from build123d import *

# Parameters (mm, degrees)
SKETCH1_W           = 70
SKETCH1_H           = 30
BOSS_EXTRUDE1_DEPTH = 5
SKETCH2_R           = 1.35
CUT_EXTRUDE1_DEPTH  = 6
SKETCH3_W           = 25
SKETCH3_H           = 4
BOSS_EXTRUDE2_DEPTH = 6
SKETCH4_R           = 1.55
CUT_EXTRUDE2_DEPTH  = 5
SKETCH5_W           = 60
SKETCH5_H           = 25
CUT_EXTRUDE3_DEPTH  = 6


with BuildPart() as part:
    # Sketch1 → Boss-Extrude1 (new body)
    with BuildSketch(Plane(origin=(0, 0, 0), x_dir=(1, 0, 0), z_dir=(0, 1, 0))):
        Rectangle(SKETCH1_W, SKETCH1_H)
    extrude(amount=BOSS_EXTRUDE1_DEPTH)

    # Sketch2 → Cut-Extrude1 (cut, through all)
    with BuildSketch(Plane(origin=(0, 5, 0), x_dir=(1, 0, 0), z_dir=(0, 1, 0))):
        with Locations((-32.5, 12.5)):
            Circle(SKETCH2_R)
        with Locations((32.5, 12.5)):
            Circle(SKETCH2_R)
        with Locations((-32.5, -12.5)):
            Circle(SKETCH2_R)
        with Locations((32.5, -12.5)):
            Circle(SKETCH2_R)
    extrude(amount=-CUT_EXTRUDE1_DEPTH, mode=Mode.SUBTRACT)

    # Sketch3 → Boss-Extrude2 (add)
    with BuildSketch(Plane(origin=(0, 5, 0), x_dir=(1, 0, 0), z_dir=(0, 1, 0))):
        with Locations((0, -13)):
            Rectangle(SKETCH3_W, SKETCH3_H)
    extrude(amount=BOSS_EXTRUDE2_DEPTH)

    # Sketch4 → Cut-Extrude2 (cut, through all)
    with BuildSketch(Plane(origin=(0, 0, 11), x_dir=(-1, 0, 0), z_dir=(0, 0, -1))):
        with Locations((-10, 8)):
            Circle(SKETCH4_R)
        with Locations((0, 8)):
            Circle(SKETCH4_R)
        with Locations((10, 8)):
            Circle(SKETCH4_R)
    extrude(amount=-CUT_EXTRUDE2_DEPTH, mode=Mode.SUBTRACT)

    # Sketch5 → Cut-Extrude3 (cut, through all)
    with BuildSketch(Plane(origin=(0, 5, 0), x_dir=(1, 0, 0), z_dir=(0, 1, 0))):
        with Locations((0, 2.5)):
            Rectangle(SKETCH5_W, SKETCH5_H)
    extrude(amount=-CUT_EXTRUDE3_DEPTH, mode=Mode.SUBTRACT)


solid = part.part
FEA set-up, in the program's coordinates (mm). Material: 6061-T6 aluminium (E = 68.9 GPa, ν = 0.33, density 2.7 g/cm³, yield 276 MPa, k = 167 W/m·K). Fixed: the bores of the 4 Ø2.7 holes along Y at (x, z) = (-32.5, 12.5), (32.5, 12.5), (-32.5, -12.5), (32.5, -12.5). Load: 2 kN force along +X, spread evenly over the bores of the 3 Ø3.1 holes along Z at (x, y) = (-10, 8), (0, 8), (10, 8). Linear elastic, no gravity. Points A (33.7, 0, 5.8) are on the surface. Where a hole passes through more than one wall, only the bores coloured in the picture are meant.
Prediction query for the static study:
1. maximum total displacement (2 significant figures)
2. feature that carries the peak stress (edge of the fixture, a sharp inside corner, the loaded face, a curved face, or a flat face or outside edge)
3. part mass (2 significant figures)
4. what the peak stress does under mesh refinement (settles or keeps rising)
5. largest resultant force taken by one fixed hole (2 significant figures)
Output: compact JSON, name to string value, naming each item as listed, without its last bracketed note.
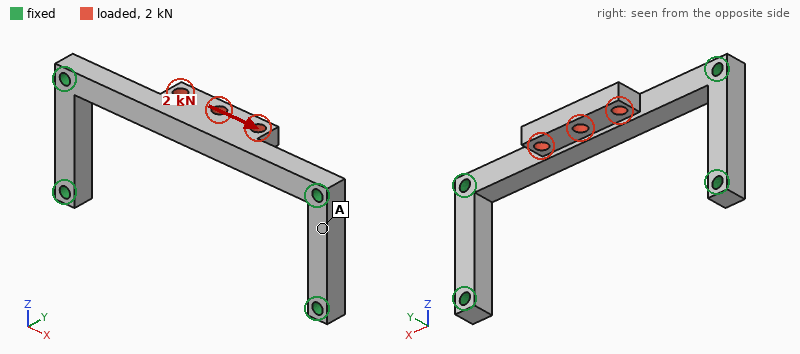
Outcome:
{"maximum total displacement": "56 µm", "feature that carries the peak stress": "edge of the fixture", "part mass": "9.2 g", "what the peak stress does under mesh refinement": "keeps rising", "largest resultant force taken by one fixed hole": "1.0 kN"}
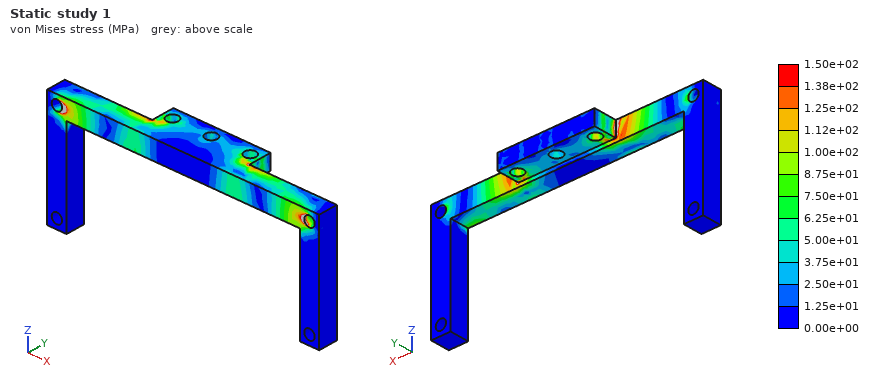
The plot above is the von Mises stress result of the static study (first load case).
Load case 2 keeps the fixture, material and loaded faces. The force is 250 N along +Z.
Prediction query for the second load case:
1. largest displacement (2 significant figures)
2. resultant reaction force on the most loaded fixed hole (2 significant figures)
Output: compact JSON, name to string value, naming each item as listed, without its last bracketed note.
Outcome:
{"largest displacement": "0.13 mm", "resultant reaction force on the most loaded fixed hole": "100 N"}
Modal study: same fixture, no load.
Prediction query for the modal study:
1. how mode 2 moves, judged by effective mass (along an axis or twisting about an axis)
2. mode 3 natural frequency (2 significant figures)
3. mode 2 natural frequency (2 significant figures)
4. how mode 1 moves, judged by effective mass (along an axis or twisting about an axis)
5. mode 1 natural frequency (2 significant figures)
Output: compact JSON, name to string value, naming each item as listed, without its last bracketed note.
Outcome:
{"how mode 2 moves, judged by effective mass": "along Y", "mode 3 natural frequency": "12 kHz", "mode 2 natural frequency": "6400 Hz", "how mode 1 moves, judged by effective mass": "along Z", "mode 1 natural frequency": "4800 Hz"}
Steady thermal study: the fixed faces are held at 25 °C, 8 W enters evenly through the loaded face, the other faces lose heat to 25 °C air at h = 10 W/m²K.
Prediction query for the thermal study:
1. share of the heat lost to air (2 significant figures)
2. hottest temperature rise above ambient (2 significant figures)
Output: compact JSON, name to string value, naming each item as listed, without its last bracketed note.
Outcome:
{"share of the heat lost to air": "3.0 %", "hottest temperature rise above ambient": "24 K"}
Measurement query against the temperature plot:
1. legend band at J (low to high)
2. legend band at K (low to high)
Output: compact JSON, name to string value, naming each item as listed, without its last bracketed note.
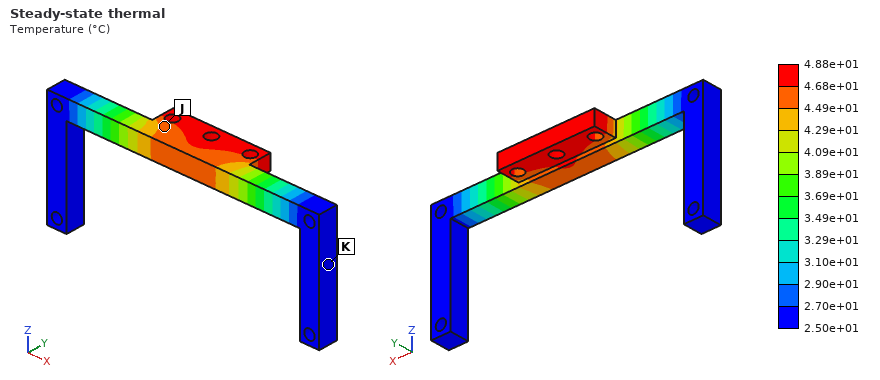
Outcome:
{"legend band at J": "4.49e+01 to 4.68e+01 °C", "legend band at K": "2.50e+01 to 2.70e+01 °C"}
